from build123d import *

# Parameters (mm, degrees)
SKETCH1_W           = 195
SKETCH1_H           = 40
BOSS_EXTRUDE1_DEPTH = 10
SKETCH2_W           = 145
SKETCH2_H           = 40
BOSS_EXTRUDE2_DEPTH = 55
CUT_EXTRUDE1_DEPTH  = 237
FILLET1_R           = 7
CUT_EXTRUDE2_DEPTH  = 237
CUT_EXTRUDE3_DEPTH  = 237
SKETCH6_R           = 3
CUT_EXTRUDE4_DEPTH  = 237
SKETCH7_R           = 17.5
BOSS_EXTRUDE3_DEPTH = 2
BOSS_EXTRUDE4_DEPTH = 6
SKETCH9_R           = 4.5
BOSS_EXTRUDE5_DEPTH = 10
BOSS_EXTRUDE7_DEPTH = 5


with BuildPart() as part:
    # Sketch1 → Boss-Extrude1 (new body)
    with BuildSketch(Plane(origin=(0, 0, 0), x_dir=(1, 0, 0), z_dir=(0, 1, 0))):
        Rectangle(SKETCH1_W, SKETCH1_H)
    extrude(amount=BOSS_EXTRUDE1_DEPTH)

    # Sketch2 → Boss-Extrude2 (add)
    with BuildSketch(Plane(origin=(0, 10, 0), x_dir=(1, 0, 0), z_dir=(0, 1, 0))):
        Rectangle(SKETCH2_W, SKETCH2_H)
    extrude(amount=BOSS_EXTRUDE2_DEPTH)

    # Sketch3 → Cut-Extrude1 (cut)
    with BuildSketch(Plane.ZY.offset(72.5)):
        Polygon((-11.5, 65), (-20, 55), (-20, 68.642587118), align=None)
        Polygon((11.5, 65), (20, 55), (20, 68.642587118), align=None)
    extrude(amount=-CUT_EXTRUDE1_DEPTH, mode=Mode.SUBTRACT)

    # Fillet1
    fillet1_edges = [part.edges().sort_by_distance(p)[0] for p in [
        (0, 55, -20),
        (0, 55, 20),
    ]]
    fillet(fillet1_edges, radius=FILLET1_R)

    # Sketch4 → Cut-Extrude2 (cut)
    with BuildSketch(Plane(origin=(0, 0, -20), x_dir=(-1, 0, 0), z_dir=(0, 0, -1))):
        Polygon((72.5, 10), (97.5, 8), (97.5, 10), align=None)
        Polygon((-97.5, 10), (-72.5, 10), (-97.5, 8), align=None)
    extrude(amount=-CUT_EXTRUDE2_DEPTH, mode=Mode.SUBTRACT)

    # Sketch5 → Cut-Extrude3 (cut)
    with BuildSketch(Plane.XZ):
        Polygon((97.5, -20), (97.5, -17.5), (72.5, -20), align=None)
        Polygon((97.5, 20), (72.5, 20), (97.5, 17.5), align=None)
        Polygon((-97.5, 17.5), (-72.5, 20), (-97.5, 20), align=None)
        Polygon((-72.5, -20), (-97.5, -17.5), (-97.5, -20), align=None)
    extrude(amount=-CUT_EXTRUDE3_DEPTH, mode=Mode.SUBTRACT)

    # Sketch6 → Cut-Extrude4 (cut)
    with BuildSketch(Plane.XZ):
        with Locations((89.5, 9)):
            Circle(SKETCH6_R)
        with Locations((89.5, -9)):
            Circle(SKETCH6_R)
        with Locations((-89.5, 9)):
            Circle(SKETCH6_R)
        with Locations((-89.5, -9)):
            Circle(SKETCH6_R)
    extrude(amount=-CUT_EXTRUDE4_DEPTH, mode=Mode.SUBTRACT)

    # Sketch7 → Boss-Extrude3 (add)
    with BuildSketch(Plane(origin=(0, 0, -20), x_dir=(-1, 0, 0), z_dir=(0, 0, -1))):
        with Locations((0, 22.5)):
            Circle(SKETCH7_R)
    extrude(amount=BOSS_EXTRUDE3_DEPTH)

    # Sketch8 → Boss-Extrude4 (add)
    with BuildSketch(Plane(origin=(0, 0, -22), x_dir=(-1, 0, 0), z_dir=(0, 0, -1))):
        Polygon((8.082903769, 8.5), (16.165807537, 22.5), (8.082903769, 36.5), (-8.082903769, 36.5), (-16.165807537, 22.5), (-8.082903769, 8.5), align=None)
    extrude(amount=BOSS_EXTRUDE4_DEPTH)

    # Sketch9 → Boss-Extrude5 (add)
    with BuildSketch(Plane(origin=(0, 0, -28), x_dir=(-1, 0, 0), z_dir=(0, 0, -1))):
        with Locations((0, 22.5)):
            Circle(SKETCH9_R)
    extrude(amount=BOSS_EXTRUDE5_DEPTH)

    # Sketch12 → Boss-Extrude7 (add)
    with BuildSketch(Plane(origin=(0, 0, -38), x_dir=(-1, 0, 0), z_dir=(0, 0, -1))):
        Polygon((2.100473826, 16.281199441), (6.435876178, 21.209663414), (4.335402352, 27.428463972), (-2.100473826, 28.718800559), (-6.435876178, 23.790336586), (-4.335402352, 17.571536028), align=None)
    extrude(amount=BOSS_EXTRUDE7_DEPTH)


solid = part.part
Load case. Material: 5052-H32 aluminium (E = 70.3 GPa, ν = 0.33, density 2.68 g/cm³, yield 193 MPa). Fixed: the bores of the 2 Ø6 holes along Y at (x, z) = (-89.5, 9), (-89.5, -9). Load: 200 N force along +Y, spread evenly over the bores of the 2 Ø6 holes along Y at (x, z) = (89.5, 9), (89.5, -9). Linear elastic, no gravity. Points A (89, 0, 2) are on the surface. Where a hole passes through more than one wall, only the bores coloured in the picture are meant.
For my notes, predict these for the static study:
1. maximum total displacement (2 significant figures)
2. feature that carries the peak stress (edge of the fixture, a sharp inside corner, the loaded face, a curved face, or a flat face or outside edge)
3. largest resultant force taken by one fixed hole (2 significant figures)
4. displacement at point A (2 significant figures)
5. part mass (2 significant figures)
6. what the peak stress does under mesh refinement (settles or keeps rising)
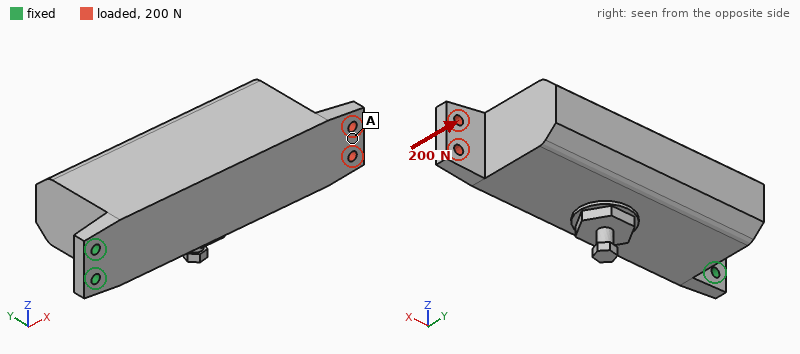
0.67 mm
edge of the fixture
110 N
0.63 mm
1.0 kg
keeps rising
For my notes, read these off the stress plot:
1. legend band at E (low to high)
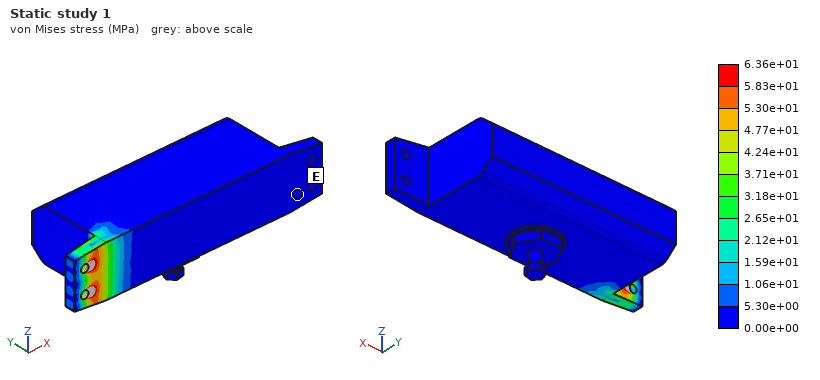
0.00e+00 to 5.30e+00 MPa
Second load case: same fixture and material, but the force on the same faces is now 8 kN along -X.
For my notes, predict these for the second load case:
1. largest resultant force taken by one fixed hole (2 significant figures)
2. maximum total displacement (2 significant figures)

4.0 kN
0.18 mm
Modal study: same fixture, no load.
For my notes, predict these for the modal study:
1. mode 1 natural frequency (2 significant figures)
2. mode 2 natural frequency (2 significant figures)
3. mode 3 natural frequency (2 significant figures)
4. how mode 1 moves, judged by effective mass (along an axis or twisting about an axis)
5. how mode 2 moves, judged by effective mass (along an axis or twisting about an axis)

160 Hz
470 Hz
990 Hz
along Y
along Z
